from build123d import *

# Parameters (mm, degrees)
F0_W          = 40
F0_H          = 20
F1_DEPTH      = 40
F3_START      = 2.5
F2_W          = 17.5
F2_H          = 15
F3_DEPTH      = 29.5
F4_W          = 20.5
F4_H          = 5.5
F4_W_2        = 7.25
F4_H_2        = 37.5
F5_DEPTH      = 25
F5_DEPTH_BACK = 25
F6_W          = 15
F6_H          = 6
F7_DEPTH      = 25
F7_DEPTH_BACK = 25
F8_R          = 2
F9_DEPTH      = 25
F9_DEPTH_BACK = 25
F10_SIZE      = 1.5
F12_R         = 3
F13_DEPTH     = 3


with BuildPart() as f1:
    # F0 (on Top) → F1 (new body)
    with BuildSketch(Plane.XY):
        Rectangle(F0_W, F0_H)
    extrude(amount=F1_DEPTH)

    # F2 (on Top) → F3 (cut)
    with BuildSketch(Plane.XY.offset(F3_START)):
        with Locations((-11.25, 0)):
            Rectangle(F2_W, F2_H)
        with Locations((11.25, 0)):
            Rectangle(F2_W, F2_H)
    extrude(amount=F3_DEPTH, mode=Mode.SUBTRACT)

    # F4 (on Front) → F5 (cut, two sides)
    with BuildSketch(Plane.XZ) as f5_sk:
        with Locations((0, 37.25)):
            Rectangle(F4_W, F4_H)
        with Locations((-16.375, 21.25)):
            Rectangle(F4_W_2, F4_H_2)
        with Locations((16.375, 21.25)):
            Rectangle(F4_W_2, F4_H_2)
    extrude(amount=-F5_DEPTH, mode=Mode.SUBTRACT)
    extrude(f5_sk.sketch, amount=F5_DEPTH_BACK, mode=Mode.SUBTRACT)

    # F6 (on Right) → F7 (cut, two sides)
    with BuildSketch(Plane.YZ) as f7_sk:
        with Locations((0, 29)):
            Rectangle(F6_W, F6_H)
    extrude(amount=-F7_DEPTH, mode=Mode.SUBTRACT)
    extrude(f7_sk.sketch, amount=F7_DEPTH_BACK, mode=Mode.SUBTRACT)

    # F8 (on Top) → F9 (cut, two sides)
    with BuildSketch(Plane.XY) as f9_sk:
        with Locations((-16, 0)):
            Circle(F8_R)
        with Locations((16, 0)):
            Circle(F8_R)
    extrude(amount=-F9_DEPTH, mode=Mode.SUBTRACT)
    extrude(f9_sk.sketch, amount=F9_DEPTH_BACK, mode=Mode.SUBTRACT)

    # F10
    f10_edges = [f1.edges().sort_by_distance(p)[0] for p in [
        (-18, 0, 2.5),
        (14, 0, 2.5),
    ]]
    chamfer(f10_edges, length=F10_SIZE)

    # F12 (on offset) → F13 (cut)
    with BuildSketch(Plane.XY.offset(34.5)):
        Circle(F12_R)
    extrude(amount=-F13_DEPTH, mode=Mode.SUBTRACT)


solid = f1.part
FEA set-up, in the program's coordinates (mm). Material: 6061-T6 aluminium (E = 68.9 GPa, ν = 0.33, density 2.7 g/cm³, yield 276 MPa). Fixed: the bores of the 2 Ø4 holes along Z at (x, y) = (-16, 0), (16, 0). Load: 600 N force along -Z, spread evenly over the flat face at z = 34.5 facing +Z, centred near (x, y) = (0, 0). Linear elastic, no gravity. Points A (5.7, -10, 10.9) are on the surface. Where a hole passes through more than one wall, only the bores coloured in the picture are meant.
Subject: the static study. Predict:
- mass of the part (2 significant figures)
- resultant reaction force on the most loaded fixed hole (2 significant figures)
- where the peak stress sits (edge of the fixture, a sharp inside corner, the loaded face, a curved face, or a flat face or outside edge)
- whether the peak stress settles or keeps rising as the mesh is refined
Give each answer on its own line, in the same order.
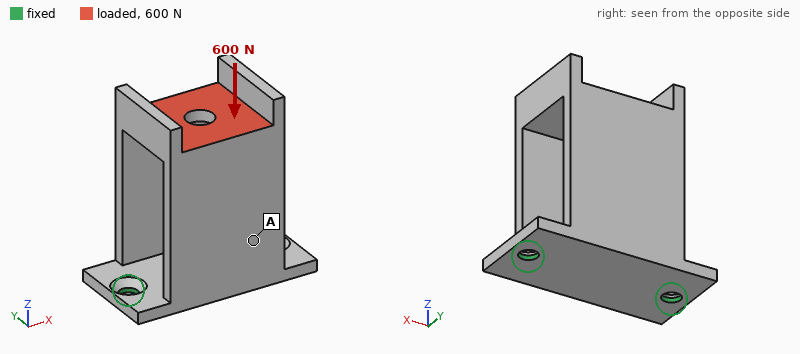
25 g
410 N
edge of the fixture
keeps rising
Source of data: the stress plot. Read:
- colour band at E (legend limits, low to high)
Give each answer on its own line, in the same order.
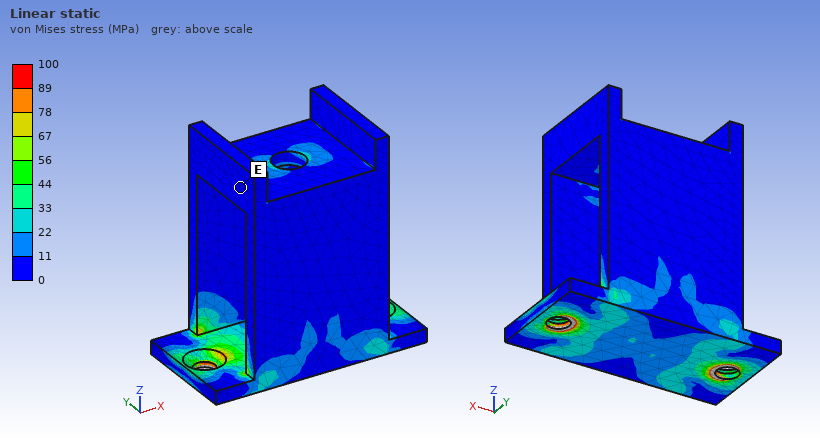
0 to 11 MPa
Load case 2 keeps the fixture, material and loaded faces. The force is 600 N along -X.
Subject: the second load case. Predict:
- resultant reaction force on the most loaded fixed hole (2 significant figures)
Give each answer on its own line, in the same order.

770 N
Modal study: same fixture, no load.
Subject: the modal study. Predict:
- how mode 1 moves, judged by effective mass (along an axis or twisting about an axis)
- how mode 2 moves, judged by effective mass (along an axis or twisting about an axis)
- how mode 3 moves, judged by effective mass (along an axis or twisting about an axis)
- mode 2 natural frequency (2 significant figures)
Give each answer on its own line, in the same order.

along Y
along X
along Z
3200 Hz
